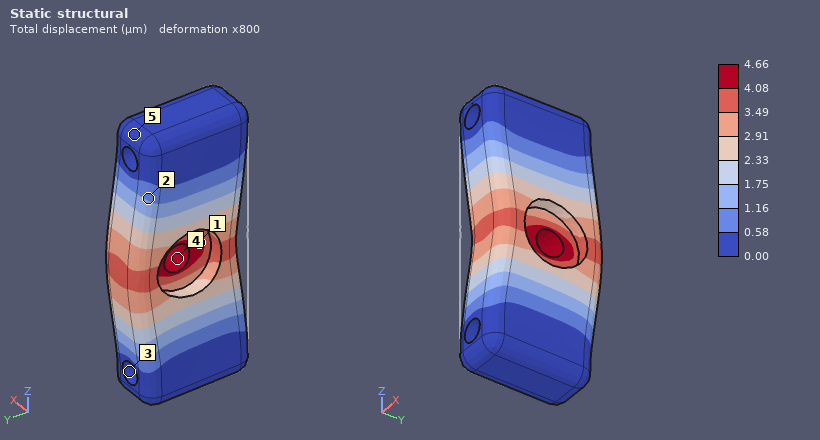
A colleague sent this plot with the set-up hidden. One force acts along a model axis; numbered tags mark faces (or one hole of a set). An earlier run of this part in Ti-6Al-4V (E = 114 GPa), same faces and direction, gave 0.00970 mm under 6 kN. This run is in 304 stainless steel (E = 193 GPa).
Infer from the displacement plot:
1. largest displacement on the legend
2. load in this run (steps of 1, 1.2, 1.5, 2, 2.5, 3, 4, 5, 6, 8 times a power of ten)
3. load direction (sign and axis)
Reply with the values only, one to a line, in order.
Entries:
4.66 µm
5 kN
+Y
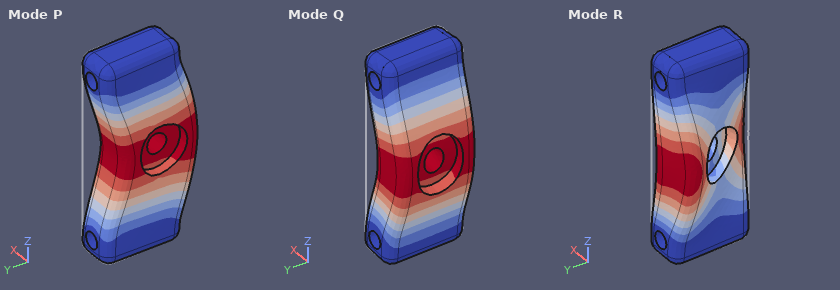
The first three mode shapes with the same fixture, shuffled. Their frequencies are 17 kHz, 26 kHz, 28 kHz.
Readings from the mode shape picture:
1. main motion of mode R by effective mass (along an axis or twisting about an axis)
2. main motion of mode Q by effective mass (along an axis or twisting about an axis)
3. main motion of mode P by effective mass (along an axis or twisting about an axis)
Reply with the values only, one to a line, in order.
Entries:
twisting about Z
along X
along Y
